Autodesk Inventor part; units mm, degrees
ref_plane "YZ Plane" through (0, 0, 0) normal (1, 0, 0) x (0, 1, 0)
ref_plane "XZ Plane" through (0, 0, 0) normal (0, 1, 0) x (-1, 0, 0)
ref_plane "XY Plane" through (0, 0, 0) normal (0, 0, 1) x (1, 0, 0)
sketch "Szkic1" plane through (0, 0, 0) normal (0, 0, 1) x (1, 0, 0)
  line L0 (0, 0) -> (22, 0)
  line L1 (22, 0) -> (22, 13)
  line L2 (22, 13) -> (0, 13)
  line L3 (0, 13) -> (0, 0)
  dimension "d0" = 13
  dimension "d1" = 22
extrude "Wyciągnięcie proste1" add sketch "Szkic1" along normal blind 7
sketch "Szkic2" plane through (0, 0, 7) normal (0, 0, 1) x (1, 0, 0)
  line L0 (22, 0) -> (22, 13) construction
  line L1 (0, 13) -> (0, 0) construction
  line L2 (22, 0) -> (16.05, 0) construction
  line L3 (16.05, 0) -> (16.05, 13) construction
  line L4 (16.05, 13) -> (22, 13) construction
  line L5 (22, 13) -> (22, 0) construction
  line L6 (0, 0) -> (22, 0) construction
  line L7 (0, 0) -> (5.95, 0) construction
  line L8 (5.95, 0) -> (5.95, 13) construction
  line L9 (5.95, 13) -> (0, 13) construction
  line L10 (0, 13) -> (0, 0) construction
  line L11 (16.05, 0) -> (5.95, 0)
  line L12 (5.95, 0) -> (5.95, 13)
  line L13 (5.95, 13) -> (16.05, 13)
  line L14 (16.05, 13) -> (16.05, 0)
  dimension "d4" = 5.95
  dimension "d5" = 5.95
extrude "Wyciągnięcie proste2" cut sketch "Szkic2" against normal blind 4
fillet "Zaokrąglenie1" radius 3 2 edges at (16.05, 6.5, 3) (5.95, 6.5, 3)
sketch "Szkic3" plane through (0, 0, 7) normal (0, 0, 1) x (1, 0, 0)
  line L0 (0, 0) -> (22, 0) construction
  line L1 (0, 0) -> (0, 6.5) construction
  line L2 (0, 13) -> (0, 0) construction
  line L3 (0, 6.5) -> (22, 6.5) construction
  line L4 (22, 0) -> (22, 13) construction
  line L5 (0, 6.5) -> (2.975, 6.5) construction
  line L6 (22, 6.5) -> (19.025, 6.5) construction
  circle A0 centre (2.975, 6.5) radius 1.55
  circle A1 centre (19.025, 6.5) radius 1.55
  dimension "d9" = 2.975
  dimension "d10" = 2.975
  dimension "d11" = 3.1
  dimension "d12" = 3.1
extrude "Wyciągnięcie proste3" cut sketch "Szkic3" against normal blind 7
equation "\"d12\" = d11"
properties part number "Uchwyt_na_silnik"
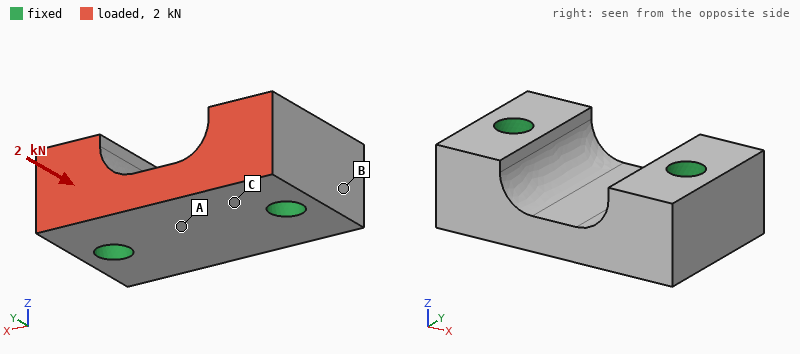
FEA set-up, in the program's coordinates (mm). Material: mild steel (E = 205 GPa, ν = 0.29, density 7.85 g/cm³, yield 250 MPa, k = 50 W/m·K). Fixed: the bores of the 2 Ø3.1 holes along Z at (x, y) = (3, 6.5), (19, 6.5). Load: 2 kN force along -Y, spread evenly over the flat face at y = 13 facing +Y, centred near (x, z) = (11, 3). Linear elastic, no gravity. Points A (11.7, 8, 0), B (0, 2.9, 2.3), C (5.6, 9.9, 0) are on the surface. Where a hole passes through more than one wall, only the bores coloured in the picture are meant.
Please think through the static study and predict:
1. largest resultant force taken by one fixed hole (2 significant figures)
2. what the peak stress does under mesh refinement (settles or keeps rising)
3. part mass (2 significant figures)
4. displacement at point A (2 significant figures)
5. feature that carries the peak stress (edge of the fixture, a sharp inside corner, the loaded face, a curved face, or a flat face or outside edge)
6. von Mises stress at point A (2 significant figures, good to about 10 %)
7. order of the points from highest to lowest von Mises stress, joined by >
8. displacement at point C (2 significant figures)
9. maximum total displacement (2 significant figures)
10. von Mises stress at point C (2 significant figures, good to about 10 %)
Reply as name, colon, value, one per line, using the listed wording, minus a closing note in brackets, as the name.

largest resultant force taken by one fixed hole: 1.0 kN
what the peak stress does under mesh refinement: keeps rising
part mass: 11 g
displacement at point A: 0.76 µm
feature that carries the peak stress: edge of the fixture
von Mises stress at point A: 9.5 MPa
order of the points from highest to lowest von Mises stress, joined by >: C > A > B
displacement at point C: 0.51 µm
maximum total displacement: 1.1 µm
von Mises stress at point C: 21 MPa
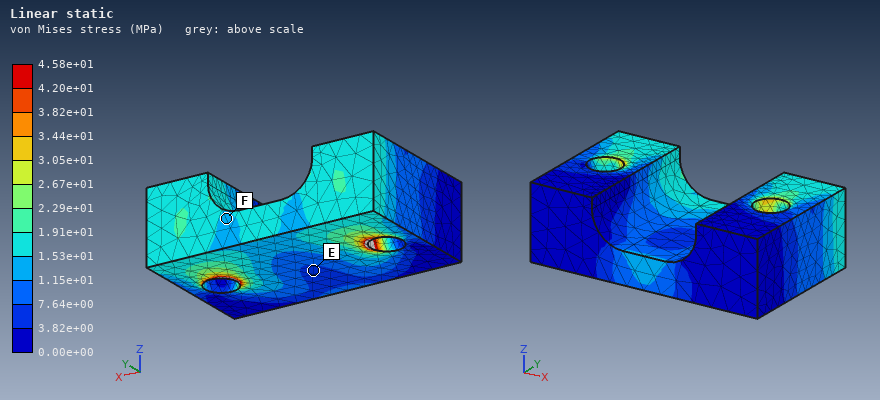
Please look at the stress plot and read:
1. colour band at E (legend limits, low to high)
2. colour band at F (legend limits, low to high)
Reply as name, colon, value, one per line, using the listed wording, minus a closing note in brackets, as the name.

colour band at E: 3.82e+00 to 7.64e+00 MPa
colour band at F: 1.15e+01 to 1.53e+01 MPa
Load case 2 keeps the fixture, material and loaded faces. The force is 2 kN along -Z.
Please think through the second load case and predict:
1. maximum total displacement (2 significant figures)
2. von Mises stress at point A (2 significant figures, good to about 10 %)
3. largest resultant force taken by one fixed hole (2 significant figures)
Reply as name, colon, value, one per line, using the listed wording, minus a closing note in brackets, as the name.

maximum total displacement: 6.2 µm
von Mises stress at point A: 39 MPa
largest resultant force taken by one fixed hole: 1.0 kN
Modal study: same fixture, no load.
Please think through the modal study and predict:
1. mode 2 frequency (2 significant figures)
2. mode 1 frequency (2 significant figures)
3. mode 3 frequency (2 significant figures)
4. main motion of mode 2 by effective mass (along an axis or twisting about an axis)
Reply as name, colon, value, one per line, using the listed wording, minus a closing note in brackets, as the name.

mode 2 frequency: 75 kHz
mode 1 frequency: 71 kHz
mode 3 frequency: 89 kHz
main motion of mode 2 by effective mass: along Z
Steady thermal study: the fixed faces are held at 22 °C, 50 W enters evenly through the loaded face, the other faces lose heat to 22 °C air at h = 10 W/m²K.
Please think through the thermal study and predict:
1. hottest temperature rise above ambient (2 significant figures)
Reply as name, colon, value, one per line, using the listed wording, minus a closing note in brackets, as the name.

hottest temperature rise above ambient: 61 K
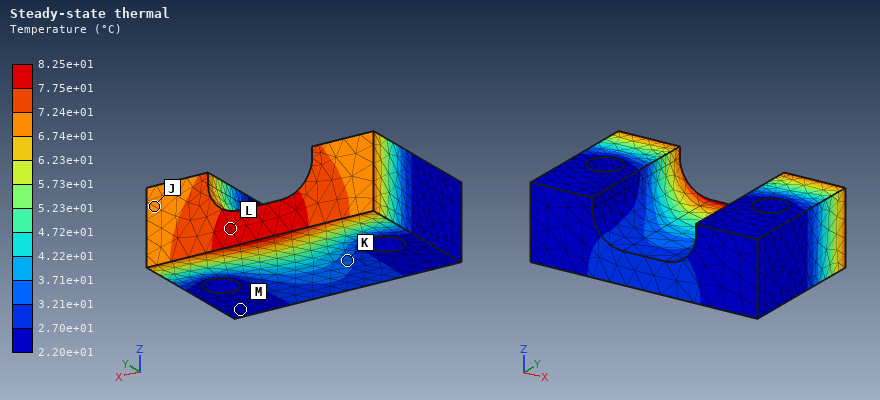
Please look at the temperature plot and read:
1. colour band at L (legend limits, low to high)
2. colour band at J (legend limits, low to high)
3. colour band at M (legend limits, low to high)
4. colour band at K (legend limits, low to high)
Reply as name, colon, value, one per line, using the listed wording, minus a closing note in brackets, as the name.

colour band at L: 7.75e+01 to 8.25e+01 °C
colour band at J: 6.74e+01 to 7.24e+01 °C
colour band at M: 2.20e+01 to 2.70e+01 °C
colour band at K: 3.21e+01 to 3.71e+01 °C
